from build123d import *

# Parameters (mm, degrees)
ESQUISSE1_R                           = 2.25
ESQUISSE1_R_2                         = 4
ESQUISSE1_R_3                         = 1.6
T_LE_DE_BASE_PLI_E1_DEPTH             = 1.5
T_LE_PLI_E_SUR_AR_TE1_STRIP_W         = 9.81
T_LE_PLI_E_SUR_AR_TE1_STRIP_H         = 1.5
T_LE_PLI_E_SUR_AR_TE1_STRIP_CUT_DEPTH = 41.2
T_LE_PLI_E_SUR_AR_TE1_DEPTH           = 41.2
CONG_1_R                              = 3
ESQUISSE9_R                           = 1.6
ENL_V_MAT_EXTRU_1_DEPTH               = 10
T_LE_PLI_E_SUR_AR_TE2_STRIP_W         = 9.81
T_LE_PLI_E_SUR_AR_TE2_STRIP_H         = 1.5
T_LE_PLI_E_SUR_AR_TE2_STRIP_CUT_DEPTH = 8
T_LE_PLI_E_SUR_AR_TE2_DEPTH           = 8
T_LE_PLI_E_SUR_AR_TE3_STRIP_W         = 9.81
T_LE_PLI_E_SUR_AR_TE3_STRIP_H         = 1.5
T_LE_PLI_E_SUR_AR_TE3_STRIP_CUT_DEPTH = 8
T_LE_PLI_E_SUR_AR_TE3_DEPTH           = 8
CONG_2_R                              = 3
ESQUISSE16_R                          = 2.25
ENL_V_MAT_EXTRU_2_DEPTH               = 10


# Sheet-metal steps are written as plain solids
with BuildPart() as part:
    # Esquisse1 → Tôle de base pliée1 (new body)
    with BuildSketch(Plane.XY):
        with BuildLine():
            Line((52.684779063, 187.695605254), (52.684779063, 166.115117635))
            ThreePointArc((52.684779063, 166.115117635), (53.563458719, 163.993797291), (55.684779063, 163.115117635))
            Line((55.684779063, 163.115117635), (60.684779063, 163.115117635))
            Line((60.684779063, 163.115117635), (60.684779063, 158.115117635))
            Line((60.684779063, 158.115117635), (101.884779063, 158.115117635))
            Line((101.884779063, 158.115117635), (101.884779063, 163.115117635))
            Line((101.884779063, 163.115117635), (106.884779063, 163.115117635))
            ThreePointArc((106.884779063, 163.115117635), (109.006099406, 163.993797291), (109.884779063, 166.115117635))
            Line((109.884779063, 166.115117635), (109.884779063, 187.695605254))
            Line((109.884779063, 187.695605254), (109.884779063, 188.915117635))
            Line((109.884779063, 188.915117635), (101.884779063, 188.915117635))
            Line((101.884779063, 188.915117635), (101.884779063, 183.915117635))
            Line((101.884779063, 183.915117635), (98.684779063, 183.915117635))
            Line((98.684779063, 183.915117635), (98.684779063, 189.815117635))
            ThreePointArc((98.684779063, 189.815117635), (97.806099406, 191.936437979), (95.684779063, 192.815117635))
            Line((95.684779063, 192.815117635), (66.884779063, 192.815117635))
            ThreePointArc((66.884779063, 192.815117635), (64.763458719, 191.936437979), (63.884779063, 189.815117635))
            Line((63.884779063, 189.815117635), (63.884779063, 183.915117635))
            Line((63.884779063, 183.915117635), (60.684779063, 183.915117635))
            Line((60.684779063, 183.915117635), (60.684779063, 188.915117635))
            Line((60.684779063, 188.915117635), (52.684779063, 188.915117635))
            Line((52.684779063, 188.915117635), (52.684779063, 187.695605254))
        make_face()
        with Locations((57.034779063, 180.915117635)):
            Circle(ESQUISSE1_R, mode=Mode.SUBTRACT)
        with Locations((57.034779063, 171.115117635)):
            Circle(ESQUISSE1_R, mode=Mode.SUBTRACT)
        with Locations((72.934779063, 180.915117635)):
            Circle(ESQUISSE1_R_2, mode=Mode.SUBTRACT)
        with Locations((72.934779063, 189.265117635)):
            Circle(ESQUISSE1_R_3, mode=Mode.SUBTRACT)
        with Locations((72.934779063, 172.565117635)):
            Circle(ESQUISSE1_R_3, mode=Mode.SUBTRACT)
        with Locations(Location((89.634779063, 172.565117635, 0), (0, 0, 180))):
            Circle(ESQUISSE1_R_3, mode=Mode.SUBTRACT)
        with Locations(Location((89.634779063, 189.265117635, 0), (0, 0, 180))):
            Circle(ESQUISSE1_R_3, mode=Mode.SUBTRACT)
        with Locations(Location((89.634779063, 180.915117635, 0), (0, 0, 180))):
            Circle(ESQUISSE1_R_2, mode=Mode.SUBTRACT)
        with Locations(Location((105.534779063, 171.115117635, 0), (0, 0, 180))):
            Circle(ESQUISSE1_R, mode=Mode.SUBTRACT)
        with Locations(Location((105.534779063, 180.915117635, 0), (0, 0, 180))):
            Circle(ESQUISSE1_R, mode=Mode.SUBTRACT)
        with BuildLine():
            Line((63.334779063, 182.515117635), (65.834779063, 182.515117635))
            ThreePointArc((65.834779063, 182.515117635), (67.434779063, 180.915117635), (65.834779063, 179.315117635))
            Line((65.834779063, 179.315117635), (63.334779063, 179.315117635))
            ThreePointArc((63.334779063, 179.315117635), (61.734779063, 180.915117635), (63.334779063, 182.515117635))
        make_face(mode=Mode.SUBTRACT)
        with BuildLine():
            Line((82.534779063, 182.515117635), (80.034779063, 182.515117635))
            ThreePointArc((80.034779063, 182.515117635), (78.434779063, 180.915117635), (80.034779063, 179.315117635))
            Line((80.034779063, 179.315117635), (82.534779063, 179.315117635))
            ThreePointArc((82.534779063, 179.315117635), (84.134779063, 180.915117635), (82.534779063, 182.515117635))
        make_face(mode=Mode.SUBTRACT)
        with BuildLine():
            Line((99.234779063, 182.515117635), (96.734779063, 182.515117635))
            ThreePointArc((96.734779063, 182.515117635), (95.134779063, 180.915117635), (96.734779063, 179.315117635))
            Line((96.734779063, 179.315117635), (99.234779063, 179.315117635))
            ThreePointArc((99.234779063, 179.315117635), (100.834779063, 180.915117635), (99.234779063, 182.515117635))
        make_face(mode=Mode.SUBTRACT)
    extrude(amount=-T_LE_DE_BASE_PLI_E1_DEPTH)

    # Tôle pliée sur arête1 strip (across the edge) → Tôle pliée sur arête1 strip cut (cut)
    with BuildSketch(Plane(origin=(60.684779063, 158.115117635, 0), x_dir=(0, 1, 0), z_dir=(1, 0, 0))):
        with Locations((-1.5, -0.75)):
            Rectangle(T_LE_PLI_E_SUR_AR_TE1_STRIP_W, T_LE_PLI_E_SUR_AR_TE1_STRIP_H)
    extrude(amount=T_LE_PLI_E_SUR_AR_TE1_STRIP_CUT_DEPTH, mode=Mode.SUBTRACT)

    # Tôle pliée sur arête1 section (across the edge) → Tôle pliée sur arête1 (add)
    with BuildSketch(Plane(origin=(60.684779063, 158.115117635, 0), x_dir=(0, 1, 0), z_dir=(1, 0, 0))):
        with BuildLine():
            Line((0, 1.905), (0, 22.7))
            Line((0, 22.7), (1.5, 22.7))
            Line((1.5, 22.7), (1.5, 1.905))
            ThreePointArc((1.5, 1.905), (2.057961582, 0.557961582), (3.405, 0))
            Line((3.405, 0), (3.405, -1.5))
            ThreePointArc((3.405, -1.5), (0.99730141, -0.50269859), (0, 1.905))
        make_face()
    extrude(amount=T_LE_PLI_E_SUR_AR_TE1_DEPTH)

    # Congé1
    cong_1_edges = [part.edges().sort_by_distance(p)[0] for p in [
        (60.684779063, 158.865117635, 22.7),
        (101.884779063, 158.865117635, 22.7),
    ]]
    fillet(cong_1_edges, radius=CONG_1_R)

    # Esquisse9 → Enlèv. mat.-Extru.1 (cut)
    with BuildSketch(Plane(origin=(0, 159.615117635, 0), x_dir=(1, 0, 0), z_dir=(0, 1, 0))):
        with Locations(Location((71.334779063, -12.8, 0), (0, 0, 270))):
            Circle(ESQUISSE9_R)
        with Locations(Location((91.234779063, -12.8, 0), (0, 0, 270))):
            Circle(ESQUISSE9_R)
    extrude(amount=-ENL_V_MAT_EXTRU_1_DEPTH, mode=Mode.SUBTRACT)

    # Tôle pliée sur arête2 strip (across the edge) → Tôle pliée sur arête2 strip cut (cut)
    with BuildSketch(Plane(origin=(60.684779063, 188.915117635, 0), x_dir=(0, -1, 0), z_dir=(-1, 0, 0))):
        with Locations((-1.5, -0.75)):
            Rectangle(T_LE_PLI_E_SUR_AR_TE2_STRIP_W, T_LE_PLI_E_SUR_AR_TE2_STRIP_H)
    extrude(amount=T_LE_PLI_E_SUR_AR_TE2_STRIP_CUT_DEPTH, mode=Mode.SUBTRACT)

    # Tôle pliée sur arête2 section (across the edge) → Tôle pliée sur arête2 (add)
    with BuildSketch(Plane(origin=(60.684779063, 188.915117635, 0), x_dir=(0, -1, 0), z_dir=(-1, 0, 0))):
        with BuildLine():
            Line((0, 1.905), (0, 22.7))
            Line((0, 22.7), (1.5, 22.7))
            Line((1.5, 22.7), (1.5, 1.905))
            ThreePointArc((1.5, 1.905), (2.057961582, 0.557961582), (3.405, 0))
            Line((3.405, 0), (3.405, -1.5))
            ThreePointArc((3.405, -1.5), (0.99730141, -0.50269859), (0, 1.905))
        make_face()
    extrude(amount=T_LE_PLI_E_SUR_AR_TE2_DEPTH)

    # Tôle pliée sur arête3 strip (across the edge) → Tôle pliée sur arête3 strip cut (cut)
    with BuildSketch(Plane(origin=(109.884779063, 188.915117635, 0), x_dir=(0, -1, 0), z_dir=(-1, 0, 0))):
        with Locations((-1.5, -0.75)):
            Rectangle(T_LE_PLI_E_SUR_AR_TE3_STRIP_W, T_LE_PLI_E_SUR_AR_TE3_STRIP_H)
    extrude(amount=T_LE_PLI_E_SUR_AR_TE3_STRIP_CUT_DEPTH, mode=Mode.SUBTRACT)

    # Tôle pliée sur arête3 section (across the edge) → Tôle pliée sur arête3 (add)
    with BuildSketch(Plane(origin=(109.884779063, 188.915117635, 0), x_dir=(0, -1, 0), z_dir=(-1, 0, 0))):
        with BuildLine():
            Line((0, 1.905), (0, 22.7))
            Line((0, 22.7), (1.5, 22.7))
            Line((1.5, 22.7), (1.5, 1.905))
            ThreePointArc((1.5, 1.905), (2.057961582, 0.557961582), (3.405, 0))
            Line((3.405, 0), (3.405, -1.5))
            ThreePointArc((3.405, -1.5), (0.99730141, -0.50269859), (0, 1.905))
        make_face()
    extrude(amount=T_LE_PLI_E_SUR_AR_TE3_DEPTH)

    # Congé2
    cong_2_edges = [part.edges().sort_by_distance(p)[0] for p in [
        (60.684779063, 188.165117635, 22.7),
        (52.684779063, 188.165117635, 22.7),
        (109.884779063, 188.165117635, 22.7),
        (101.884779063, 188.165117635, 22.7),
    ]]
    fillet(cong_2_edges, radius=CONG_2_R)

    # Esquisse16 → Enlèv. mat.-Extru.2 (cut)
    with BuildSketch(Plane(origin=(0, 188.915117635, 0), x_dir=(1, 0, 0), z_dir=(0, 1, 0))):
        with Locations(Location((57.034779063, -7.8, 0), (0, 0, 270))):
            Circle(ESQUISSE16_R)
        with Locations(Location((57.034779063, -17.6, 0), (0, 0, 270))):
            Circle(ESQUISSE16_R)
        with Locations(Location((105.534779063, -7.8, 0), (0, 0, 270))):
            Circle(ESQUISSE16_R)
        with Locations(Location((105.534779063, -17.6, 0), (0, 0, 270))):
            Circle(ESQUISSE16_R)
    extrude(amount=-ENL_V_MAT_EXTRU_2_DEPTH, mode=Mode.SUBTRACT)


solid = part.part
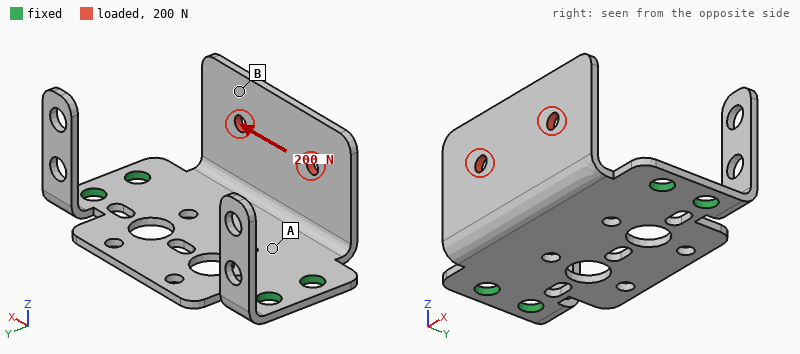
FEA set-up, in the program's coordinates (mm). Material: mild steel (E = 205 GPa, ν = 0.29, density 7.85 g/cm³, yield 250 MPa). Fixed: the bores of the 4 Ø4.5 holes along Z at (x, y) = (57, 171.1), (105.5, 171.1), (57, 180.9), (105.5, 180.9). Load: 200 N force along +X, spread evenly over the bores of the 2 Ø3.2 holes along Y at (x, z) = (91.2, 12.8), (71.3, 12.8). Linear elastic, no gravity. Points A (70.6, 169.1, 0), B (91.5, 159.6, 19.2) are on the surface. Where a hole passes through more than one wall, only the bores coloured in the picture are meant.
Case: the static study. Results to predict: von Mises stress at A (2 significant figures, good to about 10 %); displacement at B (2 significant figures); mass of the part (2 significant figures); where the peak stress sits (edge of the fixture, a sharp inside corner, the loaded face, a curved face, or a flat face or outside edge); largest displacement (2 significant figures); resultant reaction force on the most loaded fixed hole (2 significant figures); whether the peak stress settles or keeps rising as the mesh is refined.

25 MPa
39 µm
32 g
edge of the fixture
56 µm
120 N
keeps rising
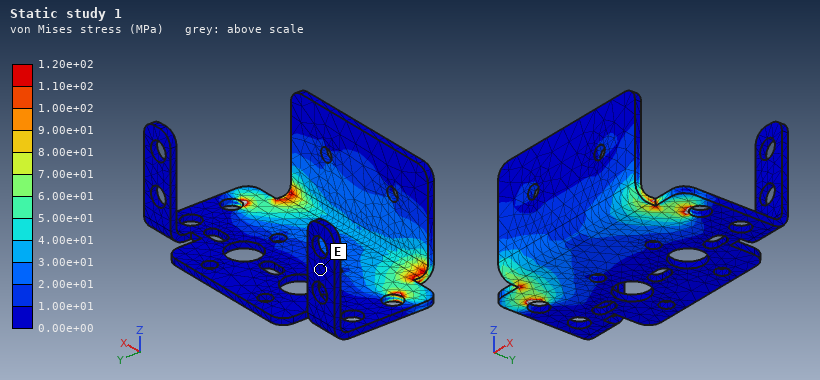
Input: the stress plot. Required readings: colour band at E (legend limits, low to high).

0.00e+00 to 1.00e+01 MPa
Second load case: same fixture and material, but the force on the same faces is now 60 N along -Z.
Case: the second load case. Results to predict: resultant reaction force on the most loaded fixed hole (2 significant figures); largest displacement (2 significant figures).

42 N
51 µm
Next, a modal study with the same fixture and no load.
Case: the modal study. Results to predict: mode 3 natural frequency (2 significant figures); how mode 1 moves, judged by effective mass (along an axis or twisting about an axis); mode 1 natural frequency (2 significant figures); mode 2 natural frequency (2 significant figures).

1900 Hz
along Y
1300 Hz
1900 Hz
